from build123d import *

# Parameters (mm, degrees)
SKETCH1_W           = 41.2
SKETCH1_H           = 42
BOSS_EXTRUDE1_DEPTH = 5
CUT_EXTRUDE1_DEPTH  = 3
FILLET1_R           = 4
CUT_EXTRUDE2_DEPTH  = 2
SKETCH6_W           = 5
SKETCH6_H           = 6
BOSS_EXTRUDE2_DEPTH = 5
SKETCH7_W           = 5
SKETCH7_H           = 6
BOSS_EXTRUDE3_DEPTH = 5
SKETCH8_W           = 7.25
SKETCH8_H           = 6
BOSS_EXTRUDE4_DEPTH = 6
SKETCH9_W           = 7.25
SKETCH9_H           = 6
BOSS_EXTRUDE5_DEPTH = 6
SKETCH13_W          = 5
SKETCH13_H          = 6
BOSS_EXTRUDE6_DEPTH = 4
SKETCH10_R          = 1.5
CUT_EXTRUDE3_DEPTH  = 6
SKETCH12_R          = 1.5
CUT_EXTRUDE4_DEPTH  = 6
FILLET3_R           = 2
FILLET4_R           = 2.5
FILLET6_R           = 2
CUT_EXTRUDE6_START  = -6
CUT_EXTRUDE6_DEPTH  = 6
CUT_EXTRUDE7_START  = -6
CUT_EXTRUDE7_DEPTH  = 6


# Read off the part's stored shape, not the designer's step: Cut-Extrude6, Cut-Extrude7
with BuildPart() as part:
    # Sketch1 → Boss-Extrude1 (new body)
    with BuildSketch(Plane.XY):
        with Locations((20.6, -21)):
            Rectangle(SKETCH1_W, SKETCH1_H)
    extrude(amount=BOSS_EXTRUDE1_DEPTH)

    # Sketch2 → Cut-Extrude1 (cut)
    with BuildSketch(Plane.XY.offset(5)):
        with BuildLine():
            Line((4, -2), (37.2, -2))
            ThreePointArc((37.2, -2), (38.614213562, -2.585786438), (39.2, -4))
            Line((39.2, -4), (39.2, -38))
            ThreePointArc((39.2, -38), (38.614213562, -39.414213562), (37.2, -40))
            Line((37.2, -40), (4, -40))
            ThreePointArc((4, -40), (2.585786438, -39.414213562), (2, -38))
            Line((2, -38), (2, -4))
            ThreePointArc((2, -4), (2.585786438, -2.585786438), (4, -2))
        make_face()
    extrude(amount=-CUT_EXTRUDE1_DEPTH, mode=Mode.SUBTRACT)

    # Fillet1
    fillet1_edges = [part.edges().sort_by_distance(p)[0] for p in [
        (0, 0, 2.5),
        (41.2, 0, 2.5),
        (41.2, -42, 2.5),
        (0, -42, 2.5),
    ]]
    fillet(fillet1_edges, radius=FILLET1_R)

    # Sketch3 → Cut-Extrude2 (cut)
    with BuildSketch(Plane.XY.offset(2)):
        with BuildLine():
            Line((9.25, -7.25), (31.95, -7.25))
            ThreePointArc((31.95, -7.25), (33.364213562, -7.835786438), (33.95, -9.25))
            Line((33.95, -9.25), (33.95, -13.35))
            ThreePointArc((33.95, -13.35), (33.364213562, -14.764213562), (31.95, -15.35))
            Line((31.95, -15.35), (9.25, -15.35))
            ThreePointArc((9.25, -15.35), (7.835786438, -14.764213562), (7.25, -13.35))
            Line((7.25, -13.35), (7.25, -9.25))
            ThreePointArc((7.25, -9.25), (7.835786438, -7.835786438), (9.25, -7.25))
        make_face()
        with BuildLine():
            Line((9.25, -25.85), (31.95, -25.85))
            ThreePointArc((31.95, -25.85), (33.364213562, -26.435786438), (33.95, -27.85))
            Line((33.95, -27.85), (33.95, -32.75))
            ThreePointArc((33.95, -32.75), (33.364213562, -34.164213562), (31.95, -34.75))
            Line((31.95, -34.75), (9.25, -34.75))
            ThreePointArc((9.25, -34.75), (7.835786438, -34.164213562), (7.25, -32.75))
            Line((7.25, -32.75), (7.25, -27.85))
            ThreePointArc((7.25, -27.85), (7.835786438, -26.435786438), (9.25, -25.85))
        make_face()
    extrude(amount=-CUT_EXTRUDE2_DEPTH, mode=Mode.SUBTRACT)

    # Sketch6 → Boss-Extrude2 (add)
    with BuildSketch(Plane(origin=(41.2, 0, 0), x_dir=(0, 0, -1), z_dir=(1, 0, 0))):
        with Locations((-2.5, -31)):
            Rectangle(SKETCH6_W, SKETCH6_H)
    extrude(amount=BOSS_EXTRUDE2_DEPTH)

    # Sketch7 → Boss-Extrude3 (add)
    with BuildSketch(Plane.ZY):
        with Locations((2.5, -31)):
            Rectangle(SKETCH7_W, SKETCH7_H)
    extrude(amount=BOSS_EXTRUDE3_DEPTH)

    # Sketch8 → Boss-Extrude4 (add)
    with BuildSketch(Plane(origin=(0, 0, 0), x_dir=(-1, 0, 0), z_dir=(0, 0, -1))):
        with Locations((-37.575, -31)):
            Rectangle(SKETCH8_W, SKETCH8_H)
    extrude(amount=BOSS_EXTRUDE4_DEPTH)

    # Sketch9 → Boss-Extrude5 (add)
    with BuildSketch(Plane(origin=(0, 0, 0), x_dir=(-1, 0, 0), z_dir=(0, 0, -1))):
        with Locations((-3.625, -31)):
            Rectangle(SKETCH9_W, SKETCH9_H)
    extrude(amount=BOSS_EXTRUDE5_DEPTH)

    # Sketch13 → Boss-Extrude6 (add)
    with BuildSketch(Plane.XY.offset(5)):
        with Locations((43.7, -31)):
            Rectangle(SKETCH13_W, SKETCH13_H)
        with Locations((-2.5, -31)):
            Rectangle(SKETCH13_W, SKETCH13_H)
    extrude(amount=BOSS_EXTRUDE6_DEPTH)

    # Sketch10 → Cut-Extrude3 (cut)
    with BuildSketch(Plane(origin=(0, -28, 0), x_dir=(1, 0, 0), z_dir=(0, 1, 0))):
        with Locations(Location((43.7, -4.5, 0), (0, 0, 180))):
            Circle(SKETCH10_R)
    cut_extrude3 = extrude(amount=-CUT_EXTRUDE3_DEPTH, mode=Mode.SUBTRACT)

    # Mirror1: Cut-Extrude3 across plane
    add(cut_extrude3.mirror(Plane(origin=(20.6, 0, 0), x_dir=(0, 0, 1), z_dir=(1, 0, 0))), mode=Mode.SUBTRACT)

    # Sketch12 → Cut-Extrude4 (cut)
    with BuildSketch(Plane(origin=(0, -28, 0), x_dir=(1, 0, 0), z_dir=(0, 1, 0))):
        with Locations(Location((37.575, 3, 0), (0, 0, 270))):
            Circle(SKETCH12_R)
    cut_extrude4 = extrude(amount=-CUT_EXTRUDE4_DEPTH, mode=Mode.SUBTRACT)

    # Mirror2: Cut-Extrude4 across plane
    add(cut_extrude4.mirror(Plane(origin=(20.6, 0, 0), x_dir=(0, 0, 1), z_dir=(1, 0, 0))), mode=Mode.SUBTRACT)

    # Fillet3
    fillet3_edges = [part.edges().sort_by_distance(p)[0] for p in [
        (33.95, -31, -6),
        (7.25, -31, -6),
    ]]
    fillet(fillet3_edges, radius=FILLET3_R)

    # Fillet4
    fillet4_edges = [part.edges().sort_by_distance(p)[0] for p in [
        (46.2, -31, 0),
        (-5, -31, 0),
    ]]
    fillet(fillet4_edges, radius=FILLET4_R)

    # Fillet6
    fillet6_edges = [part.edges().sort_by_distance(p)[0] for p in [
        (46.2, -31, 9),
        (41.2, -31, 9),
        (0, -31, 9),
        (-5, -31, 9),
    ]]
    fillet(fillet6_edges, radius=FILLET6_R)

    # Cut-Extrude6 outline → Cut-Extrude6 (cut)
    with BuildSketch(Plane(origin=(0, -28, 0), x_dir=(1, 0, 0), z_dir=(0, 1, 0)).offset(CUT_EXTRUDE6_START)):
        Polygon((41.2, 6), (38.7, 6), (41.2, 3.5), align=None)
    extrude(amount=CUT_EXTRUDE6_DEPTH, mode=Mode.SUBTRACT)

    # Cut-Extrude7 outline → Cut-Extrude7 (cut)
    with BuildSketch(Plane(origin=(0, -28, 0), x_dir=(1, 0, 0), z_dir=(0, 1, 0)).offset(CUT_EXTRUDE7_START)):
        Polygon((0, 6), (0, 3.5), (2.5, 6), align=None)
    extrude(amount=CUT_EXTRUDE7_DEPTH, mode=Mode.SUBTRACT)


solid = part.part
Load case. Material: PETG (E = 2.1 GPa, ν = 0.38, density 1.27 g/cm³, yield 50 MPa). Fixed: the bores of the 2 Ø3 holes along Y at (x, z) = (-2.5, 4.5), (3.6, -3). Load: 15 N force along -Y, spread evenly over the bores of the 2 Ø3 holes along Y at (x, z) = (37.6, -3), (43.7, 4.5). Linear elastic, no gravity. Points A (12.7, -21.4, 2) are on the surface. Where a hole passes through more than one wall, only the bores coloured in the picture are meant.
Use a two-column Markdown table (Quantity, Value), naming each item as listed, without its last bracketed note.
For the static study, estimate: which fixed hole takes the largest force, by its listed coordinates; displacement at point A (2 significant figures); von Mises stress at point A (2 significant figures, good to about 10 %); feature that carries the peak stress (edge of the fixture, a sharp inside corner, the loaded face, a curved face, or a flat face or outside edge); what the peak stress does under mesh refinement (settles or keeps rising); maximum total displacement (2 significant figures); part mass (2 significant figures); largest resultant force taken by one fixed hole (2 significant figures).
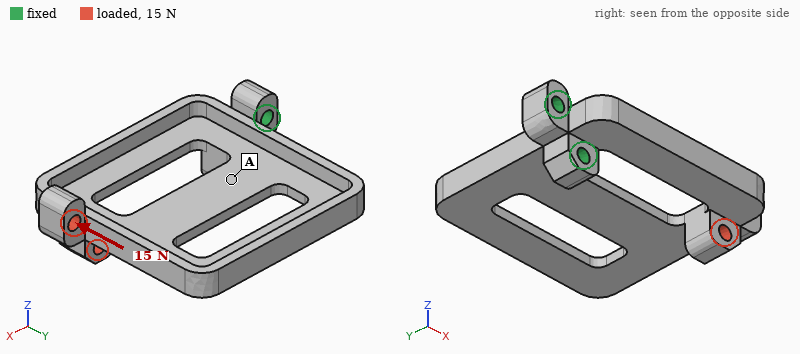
| Quantity | Value |
|---|---|
| which fixed hole takes the largest force, by its listed coordinates | (3.6, -3) |
| displacement at point A | 0.16 mm |
| von Mises stress at point A | 1.8 MPa |
| feature that carries the peak stress | a sharp inside corner |
| what the peak stress does under mesh refinement | keeps rising |
| maximum total displacement | 0.65 mm |
| part mass | 5.4 g |
| largest resultant force taken by one fixed hole | 53 N |
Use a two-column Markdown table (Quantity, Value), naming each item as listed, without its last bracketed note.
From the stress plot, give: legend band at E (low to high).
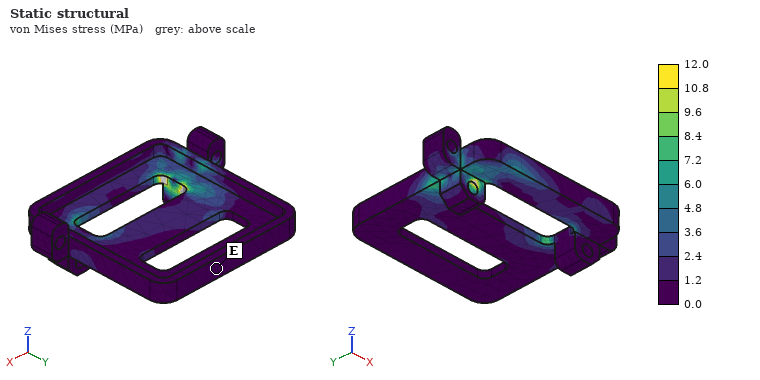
| Quantity | Value |
|---|---|
| legend band at E | 0.0 to 1.2 MPa |
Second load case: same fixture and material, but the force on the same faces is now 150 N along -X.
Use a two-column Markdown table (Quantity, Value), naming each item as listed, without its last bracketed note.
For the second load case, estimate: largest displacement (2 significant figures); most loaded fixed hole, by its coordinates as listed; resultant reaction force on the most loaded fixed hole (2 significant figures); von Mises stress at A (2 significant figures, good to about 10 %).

| Quantity | Value |
|---|---|
| largest displacement | 0.65 mm |
| most loaded fixed hole, by its coordinates as listed | (-2.5, 4.5) |
| resultant reaction force on the most loaded fixed hole | 86 N |
| von Mises stress at A | 3.1 MPa |
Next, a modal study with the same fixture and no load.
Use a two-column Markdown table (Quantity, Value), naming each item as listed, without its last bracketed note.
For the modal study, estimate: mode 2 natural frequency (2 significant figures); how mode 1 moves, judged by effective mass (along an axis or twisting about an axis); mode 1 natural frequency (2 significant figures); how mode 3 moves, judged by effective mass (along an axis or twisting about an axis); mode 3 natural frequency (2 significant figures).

| Quantity | Value |
|---|---|
| mode 2 natural frequency | 380 Hz |
| how mode 1 moves, judged by effective mass | along Z |
| mode 1 natural frequency | 190 Hz |
| how mode 3 moves, judged by effective mass | along Y |
| mode 3 natural frequency | 560 Hz |
